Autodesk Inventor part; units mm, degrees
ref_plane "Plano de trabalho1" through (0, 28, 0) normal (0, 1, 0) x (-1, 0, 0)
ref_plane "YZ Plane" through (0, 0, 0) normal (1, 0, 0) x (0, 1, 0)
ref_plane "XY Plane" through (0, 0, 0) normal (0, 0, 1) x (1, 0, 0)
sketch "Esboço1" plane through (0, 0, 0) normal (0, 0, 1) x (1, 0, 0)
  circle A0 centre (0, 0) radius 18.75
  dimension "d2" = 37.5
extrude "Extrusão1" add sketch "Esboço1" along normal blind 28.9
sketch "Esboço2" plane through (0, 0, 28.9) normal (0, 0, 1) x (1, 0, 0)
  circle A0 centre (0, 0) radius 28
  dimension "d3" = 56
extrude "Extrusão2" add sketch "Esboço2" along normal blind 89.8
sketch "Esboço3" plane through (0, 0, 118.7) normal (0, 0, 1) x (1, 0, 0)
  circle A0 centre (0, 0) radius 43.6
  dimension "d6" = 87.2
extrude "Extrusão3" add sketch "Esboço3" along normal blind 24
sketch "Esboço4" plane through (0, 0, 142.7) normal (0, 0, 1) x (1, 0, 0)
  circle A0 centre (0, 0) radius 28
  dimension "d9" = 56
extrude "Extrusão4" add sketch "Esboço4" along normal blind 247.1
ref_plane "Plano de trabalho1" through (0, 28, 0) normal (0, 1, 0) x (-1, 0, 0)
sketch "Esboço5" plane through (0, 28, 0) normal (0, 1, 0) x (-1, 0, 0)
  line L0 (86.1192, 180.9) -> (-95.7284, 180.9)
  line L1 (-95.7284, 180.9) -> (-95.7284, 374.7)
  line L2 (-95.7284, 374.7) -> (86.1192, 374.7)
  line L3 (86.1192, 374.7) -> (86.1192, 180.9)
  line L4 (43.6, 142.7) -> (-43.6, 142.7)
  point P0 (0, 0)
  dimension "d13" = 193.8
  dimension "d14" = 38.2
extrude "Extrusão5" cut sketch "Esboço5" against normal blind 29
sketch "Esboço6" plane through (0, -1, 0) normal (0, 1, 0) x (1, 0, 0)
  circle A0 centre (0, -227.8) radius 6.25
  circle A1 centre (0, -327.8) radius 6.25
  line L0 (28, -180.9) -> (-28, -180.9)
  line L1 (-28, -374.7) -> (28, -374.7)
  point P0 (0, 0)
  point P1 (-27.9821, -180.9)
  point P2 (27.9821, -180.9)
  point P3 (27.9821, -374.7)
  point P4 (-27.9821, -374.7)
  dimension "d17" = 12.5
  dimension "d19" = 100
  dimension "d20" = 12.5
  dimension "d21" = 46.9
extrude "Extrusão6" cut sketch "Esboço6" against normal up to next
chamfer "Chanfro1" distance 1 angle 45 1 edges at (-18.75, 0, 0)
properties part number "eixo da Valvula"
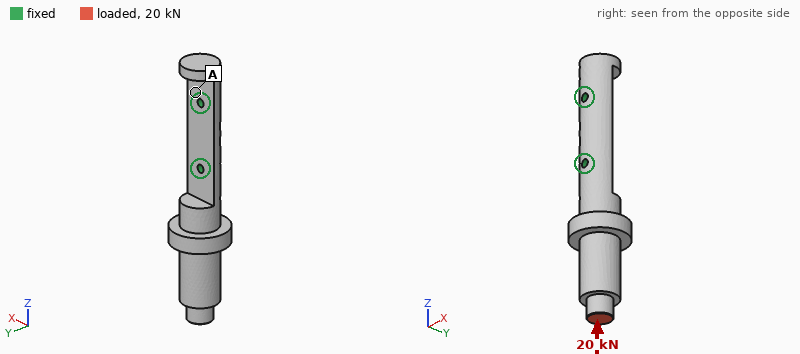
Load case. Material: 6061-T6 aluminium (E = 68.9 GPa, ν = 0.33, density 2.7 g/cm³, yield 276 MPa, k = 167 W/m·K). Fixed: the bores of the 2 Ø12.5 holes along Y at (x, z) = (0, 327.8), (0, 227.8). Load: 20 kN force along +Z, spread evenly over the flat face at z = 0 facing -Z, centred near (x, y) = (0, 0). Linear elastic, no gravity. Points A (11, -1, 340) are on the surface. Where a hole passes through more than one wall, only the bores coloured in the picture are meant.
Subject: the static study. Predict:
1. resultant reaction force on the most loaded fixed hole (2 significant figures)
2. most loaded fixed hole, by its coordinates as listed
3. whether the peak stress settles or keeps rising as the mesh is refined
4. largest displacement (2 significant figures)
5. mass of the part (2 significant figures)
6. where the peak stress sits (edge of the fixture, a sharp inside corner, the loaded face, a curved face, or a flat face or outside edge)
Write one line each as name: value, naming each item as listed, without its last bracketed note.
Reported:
resultant reaction force on the most loaded fixed hole: 18 kN
most loaded fixed hole, by its coordinates as listed: (0, 227.8)
whether the peak stress settles or keeps rising as the mesh is refined: keeps rising
largest displacement: 0.71 mm
mass of the part: 2.0 kg
where the peak stress sits: edge of the fixture
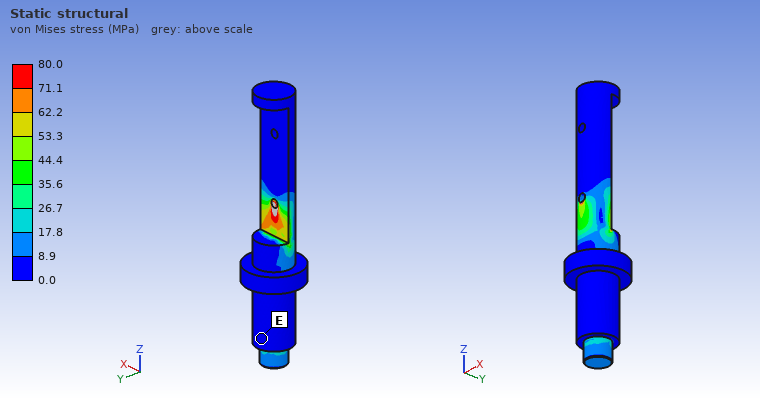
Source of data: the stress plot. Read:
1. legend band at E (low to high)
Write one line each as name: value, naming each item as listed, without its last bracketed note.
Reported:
legend band at E: 0.0 to 8.9 MPa
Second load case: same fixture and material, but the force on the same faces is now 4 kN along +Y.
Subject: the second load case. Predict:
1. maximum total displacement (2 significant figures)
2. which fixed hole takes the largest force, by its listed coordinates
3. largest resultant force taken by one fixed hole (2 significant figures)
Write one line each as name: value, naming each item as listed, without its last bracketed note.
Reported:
maximum total displacement: 2.4 mm
which fixed hole takes the largest force, by its listed coordinates: (0, 227.8)
largest resultant force taken by one fixed hole: 5.7 kN
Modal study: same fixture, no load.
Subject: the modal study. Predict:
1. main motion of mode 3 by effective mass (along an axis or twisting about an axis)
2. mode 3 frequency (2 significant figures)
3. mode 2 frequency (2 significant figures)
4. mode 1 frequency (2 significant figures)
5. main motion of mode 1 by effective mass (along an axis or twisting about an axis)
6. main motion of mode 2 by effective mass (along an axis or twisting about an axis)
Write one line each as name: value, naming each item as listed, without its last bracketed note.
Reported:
main motion of mode 3 by effective mass: twisting about Z
mode 3 frequency: 1600 Hz
mode 2 frequency: 500 Hz
mode 1 frequency: 330 Hz
main motion of mode 1 by effective mass: along Y
main motion of mode 2 by effective mass: along X
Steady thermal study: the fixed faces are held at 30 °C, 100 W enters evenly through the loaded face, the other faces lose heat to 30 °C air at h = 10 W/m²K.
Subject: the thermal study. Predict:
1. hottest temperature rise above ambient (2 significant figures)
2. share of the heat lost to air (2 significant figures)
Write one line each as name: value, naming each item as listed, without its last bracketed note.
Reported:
hottest temperature rise above ambient: 72 K
share of the heat lost to air: 17 %
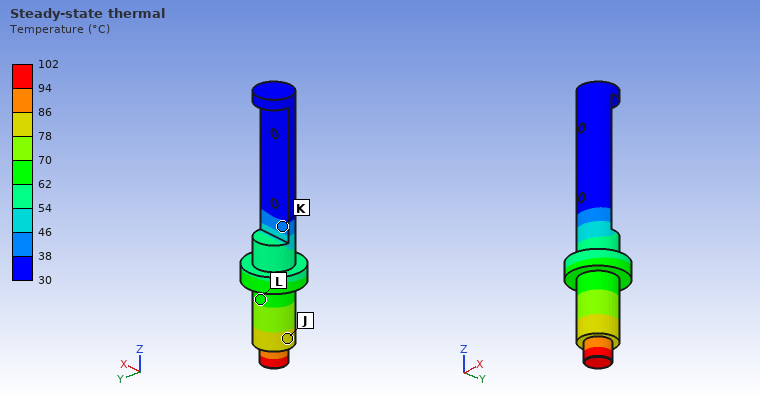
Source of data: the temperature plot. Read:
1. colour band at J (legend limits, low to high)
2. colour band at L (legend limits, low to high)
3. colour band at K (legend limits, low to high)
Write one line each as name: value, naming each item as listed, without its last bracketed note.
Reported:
colour band at J: 78 to 86 °C
colour band at L: 62 to 70 °C
colour band at K: 38 to 46 °C
